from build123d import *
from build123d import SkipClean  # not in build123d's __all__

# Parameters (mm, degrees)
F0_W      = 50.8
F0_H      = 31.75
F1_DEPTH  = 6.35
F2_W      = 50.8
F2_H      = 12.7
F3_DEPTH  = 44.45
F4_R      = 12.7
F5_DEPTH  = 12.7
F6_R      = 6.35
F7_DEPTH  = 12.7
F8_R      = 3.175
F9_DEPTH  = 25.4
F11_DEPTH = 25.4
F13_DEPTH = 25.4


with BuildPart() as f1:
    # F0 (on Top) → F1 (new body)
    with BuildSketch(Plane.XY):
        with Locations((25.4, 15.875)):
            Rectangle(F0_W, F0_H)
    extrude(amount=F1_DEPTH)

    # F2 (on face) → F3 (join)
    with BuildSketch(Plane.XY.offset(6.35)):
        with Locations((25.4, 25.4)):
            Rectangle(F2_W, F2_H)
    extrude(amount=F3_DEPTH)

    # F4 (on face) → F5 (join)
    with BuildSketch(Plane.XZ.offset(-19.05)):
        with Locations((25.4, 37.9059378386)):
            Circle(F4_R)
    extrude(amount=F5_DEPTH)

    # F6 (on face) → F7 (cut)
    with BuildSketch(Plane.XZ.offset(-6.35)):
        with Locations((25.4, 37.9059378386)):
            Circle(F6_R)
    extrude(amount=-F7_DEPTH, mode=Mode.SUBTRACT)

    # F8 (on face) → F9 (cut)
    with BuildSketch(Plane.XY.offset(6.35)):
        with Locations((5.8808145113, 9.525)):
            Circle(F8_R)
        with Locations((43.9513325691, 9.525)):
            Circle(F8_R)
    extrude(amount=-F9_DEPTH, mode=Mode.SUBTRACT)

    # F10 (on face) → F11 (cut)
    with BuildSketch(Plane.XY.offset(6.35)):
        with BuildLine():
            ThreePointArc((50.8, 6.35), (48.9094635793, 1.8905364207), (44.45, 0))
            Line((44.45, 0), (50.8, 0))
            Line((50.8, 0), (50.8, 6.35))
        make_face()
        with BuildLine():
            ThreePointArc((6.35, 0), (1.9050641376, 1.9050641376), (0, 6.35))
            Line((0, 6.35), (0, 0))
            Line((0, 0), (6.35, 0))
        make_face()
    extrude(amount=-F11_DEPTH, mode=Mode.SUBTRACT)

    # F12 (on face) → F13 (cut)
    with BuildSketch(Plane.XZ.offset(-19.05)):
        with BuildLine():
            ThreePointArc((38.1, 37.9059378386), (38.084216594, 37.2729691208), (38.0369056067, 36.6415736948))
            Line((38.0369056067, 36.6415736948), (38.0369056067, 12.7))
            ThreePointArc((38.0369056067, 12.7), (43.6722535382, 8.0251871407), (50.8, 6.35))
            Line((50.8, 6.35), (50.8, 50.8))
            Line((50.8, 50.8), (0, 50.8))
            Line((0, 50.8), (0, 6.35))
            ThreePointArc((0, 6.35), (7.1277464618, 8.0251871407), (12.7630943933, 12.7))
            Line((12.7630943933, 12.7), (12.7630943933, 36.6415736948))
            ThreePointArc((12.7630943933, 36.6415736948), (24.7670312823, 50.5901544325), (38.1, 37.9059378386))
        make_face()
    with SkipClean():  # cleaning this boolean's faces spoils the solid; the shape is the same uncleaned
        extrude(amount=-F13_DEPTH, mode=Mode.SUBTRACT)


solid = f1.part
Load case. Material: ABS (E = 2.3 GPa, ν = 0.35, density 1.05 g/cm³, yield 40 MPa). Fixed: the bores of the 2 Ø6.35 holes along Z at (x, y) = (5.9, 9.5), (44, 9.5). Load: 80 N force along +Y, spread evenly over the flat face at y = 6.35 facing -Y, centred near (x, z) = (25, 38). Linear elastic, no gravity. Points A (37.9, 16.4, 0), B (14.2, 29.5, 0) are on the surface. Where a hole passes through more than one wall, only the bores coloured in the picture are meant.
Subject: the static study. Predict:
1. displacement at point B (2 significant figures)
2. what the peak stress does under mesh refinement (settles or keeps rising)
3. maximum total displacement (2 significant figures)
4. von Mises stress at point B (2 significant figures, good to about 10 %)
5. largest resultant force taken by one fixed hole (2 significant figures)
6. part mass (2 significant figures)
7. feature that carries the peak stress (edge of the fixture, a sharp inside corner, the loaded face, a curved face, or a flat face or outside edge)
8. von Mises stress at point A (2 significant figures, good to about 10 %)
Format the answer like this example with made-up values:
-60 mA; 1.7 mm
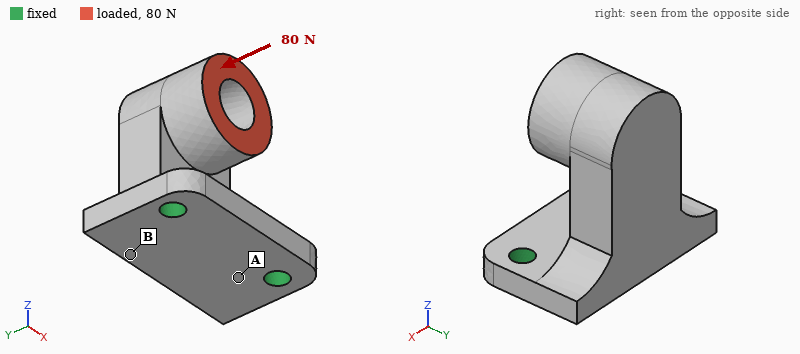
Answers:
0.20 mm; keeps rising; 0.87 mm; 1.9 MPa; 45 N; 30 g; edge of the fixture; 6.8 MPa
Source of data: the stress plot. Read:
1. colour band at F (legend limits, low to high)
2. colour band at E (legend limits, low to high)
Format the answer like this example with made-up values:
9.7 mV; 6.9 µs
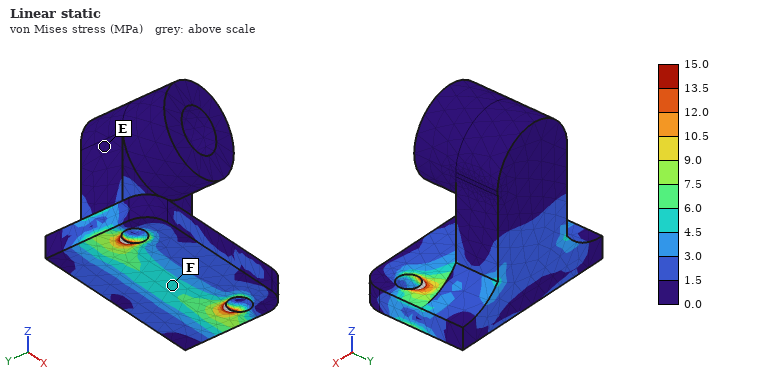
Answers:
4.5 to 6.0 MPa; 0.0 to 1.5 MPa
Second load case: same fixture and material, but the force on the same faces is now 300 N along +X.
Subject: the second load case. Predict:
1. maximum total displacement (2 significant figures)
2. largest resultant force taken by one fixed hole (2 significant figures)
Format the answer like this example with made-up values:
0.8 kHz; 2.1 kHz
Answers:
0.90 mm; 330 N
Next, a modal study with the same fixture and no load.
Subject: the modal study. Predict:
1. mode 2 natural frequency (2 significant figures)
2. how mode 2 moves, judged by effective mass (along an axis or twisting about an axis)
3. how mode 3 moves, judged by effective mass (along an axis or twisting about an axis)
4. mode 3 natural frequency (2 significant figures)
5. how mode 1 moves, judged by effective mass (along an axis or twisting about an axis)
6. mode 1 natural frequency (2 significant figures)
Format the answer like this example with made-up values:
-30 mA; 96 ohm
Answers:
1100 Hz; along X; along Z; 1900 Hz; along Y; 470 Hz
